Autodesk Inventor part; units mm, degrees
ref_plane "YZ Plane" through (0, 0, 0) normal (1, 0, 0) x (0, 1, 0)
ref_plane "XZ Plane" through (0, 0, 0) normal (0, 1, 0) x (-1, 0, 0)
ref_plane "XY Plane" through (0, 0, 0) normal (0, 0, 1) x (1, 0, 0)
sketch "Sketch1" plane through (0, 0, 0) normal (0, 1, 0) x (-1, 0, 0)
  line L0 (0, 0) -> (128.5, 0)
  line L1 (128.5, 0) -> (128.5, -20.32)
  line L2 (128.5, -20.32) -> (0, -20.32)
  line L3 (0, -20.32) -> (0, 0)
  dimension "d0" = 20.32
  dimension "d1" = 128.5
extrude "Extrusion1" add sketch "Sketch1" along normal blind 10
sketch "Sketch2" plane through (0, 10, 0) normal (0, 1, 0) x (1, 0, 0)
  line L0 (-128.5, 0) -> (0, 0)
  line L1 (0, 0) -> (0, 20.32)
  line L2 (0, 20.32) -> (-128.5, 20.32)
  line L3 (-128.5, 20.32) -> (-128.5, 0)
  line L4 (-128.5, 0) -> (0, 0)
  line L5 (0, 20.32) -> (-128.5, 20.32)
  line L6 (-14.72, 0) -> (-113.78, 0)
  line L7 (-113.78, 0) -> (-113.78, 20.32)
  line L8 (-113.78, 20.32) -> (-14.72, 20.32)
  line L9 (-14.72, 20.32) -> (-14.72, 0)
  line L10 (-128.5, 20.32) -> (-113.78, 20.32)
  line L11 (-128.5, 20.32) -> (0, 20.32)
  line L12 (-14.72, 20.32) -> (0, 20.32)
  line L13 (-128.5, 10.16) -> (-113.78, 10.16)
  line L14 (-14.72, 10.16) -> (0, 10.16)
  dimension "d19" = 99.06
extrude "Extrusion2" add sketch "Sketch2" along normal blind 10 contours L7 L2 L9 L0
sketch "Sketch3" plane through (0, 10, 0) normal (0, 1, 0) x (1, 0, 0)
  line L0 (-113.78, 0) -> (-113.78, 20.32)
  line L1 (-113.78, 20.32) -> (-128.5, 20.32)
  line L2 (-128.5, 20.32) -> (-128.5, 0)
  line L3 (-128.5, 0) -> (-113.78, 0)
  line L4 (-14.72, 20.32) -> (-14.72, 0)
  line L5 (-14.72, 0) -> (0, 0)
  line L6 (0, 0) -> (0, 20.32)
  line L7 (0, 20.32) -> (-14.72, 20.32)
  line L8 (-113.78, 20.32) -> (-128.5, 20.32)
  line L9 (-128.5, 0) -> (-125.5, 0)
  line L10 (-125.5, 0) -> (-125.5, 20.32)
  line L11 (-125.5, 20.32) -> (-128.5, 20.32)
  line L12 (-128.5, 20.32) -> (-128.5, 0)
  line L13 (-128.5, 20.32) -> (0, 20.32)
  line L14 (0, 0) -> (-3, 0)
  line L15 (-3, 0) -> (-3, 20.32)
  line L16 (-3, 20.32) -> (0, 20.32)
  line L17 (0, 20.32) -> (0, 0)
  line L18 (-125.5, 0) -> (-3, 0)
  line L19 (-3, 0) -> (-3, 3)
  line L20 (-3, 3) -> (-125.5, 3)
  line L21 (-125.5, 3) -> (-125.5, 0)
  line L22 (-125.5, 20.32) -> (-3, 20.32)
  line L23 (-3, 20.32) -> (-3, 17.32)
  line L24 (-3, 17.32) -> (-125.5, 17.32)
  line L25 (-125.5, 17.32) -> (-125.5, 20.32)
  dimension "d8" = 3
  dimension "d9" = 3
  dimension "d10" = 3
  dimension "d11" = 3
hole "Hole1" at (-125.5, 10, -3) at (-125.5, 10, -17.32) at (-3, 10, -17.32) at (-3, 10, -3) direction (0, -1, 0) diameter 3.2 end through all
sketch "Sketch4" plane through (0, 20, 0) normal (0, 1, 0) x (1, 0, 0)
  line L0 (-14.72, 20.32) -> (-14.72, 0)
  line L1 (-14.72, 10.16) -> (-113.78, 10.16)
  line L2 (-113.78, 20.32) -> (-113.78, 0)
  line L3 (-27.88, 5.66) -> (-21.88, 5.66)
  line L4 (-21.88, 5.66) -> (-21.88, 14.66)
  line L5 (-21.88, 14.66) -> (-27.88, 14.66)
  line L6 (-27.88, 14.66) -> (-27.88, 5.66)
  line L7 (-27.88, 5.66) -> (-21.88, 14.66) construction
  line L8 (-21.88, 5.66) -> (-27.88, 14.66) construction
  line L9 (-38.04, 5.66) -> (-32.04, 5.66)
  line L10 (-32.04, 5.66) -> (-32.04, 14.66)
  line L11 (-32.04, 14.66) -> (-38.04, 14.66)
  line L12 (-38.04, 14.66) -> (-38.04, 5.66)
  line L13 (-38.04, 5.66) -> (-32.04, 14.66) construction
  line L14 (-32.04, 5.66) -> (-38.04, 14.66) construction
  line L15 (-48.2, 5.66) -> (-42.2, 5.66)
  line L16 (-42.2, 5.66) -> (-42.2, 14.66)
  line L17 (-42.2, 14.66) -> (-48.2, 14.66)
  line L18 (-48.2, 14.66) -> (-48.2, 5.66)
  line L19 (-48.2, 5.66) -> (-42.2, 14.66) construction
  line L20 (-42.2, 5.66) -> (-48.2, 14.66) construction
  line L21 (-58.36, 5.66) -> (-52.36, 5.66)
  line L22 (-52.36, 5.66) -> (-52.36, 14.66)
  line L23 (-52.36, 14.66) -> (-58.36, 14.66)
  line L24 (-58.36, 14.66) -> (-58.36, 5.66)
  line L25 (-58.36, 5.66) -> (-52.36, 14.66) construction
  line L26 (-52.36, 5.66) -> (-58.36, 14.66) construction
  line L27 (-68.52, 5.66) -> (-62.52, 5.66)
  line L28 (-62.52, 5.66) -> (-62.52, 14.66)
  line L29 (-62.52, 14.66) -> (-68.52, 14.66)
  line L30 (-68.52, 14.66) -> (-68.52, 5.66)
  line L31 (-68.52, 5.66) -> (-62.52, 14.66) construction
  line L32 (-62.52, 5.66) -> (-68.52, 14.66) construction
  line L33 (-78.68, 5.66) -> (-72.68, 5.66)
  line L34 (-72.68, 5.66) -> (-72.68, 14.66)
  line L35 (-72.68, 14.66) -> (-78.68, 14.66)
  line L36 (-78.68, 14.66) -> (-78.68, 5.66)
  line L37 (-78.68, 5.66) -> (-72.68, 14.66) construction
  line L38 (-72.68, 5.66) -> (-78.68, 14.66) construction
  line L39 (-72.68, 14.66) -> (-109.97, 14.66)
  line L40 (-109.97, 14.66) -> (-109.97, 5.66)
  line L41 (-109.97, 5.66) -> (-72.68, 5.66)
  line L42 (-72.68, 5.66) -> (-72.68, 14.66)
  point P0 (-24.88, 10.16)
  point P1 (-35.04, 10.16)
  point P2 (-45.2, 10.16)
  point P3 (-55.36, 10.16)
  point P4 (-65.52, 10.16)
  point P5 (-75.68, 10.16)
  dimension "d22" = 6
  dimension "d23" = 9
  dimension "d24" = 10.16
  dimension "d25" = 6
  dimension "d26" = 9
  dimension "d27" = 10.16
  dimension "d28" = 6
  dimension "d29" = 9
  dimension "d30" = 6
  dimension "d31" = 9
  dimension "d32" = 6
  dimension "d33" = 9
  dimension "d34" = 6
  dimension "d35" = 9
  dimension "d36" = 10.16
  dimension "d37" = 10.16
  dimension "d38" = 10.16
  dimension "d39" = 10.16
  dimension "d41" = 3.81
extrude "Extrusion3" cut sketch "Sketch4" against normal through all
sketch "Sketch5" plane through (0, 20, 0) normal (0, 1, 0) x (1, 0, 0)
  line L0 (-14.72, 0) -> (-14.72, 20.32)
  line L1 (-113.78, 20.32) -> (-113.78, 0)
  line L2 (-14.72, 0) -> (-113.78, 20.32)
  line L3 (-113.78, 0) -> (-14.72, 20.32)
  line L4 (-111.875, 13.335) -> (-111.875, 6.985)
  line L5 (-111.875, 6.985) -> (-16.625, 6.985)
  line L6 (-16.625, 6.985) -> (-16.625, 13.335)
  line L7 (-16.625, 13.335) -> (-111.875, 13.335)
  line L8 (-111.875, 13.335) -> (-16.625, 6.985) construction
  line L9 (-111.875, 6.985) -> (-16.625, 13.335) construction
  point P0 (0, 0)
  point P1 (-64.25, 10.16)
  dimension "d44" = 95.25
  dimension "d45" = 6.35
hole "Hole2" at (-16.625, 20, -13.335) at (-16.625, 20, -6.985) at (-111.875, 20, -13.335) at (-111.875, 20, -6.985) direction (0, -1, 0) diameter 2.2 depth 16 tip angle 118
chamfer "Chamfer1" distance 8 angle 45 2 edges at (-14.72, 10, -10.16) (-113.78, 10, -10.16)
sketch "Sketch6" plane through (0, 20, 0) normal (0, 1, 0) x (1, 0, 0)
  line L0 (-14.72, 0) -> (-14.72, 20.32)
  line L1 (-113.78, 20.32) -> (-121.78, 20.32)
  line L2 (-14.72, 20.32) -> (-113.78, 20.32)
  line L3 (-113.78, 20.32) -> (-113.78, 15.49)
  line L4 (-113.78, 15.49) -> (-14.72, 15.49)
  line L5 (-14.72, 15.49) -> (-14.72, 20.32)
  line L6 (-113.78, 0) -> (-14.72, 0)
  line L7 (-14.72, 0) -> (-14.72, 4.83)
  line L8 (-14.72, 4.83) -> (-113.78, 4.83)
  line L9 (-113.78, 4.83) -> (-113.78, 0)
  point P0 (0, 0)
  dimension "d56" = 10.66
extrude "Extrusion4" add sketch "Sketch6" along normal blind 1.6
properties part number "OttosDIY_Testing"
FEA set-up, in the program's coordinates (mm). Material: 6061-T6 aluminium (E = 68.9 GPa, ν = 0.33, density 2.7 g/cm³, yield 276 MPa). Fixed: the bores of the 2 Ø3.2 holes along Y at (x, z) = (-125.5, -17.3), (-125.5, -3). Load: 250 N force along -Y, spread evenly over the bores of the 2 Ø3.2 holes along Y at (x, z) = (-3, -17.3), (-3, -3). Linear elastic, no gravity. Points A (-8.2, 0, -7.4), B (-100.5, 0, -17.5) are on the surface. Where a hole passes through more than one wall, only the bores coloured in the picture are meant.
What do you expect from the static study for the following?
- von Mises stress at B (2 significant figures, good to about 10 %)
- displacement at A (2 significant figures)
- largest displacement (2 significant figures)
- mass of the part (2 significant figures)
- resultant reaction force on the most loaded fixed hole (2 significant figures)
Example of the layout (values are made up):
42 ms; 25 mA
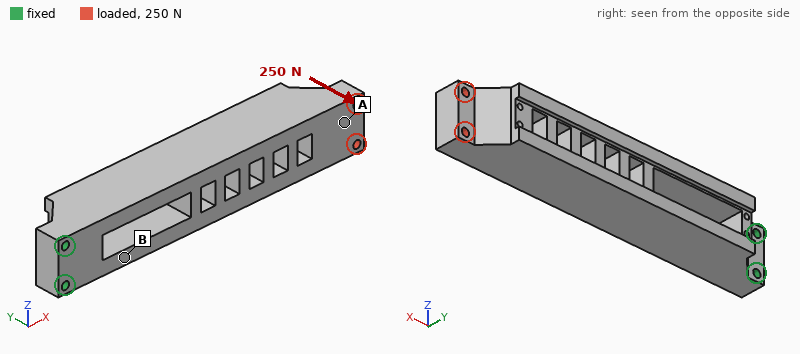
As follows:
29 MPa; 0.47 mm; 0.51 mm; 98 g; 150 N
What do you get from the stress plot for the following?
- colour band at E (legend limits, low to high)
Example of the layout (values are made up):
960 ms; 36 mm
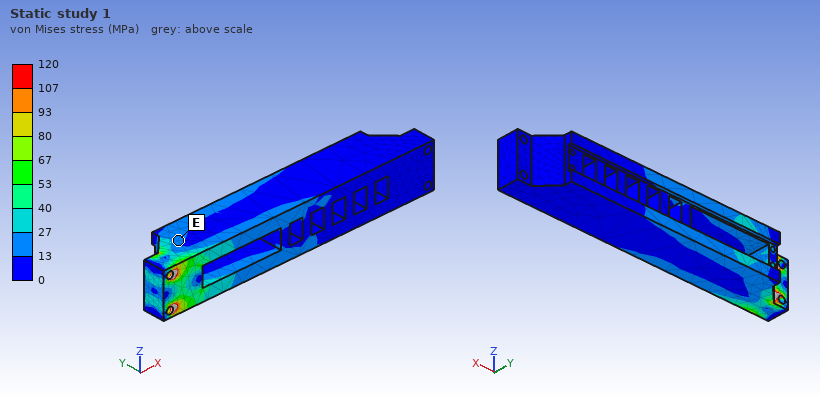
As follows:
13 to 27 MPa
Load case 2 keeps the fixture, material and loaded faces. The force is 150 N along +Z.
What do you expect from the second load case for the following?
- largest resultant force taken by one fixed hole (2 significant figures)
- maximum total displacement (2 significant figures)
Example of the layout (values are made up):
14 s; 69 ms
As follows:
1.2 kN; 0.17 mm
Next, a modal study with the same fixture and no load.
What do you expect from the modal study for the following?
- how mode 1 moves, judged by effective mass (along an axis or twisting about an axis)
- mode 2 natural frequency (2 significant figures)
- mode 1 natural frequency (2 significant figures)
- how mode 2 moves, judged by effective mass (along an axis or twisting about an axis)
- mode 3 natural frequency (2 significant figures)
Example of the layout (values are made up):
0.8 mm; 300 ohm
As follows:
along Y; 850 Hz; 650 Hz; along Z; 3000 Hz
